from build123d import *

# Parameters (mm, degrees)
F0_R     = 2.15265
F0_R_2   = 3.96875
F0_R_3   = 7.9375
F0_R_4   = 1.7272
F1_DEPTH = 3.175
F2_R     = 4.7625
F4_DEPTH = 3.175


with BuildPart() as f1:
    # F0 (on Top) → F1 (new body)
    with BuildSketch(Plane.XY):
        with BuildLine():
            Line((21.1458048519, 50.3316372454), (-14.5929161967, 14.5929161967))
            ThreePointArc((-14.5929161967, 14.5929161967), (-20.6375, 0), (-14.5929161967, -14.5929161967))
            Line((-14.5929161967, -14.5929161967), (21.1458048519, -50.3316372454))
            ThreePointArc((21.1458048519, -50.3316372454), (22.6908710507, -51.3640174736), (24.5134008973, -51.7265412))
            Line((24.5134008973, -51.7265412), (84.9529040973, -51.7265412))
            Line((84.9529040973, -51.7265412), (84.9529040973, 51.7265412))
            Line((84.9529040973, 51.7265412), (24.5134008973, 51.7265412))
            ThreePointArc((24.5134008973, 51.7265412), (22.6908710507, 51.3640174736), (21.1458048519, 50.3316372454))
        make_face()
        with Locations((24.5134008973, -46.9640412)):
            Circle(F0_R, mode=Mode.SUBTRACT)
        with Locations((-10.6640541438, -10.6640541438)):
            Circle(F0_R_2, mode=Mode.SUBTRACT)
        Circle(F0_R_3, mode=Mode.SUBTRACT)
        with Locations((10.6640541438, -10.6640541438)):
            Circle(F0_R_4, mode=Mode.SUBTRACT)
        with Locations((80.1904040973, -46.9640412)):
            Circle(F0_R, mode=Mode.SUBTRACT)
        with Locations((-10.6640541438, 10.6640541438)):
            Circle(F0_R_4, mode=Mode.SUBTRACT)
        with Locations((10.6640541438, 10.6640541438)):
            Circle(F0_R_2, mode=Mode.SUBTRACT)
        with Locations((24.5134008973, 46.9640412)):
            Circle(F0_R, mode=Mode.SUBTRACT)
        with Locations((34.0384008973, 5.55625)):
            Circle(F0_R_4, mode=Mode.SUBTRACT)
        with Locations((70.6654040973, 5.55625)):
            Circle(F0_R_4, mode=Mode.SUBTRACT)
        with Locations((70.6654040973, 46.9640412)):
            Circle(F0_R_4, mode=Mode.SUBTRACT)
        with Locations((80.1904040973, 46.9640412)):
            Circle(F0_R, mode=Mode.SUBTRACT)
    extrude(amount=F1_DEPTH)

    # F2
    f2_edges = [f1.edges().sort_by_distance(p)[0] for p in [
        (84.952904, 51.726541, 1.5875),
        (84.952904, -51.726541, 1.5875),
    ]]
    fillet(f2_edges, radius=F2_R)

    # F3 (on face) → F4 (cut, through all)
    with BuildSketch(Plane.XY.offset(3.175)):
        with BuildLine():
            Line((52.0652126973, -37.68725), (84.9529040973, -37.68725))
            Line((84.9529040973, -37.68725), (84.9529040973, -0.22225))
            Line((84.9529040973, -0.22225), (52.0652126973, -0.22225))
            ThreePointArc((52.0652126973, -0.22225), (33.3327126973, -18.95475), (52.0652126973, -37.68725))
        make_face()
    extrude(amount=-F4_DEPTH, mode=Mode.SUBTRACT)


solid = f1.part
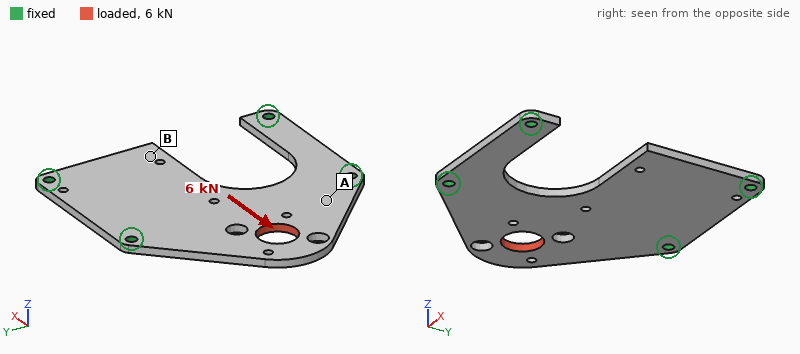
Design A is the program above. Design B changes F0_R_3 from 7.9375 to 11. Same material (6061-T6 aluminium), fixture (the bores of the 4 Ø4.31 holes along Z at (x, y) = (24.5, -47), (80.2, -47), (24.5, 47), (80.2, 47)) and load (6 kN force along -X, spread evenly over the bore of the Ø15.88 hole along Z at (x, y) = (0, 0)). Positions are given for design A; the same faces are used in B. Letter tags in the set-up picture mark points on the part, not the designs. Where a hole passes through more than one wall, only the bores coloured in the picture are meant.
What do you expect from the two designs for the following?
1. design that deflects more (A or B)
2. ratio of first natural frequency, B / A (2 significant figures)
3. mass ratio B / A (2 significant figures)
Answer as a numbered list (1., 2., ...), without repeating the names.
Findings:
1. B
2. 1.0
3. 0.97
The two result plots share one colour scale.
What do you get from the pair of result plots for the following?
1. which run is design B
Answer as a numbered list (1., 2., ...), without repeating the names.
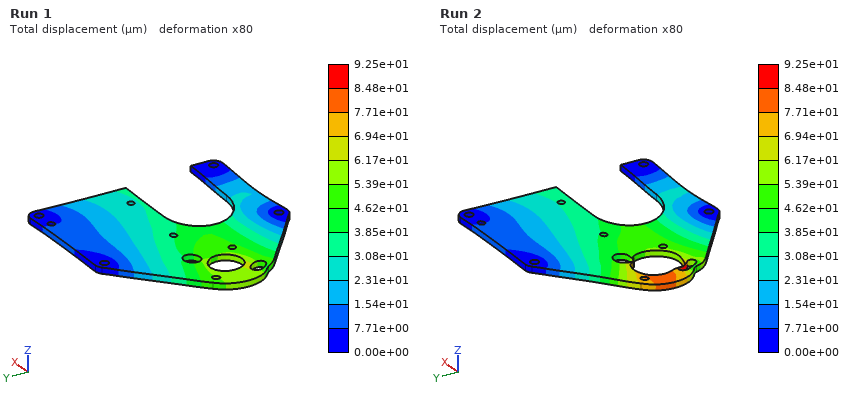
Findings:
1. Run 2
